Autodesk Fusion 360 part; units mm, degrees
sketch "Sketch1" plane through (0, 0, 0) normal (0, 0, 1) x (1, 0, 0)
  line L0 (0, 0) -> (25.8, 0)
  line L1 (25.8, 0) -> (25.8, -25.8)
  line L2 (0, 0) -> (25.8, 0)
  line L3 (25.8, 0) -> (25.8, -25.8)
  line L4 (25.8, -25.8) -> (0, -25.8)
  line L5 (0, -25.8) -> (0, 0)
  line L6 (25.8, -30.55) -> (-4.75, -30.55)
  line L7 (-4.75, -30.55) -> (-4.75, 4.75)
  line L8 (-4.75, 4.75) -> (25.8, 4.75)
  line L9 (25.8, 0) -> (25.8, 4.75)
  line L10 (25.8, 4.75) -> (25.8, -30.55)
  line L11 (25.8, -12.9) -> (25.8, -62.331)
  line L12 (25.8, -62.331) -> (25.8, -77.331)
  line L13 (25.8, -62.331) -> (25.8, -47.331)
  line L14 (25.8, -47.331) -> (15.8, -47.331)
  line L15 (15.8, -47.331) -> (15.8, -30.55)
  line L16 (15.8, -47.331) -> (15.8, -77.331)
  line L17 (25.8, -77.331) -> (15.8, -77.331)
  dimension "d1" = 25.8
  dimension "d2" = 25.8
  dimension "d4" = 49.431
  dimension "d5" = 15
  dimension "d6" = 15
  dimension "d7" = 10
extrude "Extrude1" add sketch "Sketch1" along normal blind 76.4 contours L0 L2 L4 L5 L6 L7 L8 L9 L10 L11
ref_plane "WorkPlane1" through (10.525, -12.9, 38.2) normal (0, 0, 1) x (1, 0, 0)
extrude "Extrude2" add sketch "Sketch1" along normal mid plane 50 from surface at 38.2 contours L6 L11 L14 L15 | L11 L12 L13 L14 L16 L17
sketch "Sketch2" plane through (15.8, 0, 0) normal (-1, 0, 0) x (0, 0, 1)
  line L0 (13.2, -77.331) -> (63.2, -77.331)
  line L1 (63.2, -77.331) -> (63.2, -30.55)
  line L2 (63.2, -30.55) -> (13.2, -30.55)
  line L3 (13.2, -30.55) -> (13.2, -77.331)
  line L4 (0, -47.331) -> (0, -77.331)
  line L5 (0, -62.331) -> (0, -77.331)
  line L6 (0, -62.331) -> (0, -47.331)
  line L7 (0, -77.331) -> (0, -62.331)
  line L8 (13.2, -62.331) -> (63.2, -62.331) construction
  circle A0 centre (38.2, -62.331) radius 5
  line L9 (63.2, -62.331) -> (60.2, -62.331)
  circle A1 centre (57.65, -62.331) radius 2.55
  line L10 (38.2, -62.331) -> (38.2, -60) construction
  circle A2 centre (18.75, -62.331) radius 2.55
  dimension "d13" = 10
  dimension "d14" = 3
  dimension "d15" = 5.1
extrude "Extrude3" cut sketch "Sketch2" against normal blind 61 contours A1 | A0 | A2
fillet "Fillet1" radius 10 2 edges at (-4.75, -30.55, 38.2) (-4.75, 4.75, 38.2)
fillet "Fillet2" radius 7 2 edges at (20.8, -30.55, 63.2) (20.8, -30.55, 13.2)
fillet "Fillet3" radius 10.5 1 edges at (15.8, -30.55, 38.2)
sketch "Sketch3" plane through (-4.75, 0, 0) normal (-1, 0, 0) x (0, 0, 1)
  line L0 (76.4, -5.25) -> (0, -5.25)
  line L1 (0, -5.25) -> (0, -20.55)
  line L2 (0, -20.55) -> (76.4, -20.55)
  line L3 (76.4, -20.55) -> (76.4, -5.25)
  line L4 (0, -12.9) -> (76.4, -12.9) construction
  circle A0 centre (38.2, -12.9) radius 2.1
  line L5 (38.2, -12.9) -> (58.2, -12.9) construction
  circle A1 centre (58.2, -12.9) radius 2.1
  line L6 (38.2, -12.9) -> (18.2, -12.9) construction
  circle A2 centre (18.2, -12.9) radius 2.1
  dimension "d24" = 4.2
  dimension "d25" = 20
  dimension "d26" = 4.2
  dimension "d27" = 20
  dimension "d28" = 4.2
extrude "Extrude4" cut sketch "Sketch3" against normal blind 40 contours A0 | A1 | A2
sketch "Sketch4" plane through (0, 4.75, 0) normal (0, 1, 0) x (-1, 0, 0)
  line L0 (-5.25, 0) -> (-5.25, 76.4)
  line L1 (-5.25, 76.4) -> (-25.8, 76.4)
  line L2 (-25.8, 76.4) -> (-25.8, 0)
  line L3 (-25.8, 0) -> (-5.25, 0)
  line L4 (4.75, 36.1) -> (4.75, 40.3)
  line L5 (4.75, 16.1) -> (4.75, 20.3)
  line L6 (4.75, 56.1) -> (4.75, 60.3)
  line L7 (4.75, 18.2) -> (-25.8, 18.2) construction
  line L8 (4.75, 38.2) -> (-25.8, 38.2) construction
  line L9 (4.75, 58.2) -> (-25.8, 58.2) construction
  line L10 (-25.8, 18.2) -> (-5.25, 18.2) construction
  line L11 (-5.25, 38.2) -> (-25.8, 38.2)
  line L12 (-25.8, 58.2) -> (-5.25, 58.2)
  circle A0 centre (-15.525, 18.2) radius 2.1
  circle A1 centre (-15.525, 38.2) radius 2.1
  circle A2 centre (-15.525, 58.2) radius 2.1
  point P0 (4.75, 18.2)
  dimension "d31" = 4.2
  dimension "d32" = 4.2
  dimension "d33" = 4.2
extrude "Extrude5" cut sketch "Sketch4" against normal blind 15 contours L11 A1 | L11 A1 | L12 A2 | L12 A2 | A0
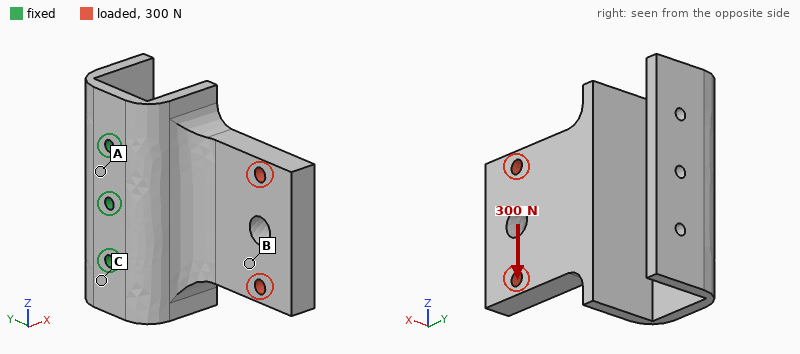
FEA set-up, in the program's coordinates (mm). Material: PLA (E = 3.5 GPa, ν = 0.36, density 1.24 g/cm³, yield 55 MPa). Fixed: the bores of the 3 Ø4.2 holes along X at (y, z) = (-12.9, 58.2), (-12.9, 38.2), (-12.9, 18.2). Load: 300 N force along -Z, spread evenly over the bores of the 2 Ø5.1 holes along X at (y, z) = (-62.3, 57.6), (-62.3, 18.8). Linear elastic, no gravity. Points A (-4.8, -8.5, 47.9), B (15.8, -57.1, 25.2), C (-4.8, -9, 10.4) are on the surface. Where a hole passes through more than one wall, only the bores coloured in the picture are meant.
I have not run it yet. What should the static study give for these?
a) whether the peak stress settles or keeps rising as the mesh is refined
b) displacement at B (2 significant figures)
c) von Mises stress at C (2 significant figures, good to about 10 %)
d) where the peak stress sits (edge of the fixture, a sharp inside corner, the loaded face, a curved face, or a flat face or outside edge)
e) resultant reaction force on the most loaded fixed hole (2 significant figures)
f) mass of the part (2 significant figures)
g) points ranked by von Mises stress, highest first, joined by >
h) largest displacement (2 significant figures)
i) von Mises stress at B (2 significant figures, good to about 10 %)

keeps rising
0.40 mm
5.1 MPa
edge of the fixture
390 N
64 g
C > B > A
0.64 mm
2.7 MPa
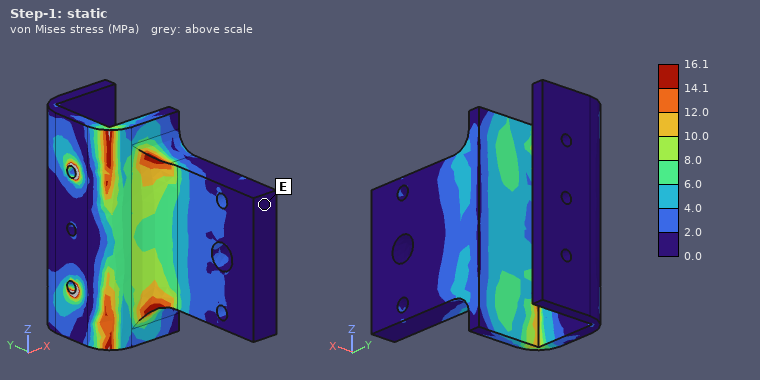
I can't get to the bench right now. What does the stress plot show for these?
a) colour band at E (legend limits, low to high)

0.0 to 2.0 MPa
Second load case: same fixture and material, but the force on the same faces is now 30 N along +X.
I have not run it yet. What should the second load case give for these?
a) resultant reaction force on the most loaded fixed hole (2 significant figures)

11 N
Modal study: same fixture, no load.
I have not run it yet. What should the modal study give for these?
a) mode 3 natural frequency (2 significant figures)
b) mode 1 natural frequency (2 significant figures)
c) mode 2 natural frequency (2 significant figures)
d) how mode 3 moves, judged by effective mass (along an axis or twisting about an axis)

820 Hz
190 Hz
760 Hz
along Z
